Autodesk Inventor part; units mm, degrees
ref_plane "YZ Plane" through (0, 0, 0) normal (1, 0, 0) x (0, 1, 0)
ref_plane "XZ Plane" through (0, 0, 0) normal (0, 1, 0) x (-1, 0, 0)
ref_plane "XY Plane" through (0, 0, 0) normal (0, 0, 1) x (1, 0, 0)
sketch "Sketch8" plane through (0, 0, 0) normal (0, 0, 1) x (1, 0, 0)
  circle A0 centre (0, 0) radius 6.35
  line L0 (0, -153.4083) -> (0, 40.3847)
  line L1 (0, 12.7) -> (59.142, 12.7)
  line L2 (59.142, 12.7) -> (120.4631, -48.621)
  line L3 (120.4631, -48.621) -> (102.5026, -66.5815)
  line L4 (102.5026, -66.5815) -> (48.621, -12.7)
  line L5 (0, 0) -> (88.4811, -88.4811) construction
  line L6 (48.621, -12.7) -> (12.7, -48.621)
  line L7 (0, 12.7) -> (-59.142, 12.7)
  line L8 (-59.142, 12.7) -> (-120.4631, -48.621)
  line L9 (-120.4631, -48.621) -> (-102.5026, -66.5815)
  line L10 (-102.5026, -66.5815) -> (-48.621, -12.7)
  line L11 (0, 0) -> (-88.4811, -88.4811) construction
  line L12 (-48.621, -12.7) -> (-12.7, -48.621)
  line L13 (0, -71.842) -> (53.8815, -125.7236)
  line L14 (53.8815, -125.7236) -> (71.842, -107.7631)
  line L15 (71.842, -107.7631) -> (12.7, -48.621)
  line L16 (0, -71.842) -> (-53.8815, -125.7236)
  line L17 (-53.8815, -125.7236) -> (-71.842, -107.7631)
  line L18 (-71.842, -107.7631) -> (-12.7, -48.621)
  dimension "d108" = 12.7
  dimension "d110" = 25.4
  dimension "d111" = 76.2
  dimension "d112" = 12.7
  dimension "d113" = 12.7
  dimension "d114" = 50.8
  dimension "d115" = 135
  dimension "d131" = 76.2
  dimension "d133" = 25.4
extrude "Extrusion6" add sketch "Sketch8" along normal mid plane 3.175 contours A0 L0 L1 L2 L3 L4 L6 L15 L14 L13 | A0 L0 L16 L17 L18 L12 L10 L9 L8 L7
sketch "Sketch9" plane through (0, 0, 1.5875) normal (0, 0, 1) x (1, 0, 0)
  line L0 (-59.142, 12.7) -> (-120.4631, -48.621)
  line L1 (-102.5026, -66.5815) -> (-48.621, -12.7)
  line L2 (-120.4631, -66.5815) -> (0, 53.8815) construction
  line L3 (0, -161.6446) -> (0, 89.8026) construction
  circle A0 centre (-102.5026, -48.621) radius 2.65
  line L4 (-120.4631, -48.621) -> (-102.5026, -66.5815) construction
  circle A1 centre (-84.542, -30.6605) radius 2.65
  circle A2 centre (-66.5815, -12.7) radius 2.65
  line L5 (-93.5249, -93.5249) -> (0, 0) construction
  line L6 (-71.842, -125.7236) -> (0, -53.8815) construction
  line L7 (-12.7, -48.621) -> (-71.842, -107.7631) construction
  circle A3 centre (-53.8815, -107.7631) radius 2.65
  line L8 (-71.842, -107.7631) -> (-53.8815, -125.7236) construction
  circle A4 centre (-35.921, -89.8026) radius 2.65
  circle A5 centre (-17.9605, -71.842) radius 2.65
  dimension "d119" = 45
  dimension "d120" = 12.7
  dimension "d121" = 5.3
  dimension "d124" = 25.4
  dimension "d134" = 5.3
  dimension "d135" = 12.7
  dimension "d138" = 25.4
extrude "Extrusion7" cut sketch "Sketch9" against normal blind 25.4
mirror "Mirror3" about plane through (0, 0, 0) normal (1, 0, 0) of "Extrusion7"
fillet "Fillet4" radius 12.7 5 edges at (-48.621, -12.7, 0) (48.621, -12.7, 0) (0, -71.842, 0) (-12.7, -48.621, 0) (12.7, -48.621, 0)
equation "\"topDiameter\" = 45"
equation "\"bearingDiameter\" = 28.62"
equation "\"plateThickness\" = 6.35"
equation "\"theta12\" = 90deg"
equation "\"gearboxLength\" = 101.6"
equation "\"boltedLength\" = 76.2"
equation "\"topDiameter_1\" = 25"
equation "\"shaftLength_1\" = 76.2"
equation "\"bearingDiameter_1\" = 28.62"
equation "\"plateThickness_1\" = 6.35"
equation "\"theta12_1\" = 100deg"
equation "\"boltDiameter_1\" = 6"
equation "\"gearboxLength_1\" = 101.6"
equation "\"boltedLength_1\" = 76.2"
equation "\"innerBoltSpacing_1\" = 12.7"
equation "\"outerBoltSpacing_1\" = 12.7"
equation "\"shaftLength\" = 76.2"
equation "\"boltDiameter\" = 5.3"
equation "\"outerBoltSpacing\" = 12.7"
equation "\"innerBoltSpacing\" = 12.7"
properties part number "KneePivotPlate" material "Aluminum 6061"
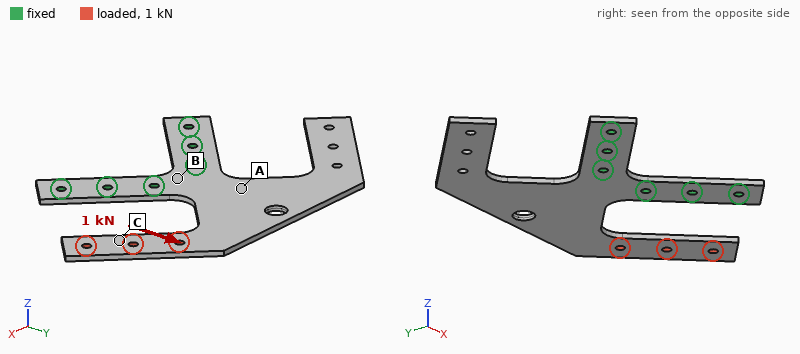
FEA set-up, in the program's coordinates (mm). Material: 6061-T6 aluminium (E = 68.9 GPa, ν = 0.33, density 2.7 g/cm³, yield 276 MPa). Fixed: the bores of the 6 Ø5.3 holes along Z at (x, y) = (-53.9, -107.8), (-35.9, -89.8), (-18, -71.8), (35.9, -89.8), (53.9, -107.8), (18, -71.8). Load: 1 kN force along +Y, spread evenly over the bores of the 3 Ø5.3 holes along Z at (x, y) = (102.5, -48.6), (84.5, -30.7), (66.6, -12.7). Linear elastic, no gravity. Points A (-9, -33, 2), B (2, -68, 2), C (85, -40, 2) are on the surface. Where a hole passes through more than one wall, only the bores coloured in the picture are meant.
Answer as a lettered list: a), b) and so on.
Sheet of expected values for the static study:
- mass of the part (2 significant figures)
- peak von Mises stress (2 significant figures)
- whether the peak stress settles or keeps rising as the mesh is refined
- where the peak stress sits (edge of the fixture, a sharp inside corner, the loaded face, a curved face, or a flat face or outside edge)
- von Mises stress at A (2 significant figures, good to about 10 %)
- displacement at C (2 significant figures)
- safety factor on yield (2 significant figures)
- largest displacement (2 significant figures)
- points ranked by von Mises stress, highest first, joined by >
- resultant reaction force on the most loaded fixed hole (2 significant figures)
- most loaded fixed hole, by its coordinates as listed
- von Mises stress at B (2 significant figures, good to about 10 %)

a) 110 g
b) 190 MPa
c) settles
d) a curved face
e) 43 MPa
f) 0.50 mm
g) 1.5
h) 0.80 mm
i) A > B > C
j) 2.4 kN
k) (18, -71.8)
l) 26 MPa
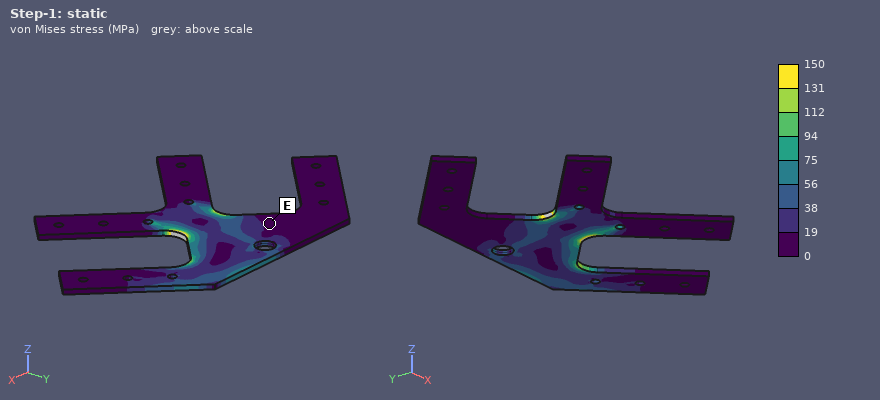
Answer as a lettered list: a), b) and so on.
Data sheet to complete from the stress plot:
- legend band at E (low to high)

a) 0 to 19 MPa
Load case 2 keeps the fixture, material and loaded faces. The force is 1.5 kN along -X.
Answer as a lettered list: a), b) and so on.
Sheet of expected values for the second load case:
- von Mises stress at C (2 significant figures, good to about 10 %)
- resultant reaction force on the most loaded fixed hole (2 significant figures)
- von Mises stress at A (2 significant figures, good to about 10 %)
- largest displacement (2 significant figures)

a) 20 MPa
b) 1.4 kN
c) 16 MPa
d) 0.35 mm
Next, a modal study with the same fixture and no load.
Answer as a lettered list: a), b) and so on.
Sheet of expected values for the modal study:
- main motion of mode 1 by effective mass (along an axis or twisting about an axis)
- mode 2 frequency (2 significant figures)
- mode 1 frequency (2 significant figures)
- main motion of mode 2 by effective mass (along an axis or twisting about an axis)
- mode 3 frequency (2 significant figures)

a) twisting about Y
b) 190 Hz
c) 150 Hz
d) along Z
e) 240 Hz
